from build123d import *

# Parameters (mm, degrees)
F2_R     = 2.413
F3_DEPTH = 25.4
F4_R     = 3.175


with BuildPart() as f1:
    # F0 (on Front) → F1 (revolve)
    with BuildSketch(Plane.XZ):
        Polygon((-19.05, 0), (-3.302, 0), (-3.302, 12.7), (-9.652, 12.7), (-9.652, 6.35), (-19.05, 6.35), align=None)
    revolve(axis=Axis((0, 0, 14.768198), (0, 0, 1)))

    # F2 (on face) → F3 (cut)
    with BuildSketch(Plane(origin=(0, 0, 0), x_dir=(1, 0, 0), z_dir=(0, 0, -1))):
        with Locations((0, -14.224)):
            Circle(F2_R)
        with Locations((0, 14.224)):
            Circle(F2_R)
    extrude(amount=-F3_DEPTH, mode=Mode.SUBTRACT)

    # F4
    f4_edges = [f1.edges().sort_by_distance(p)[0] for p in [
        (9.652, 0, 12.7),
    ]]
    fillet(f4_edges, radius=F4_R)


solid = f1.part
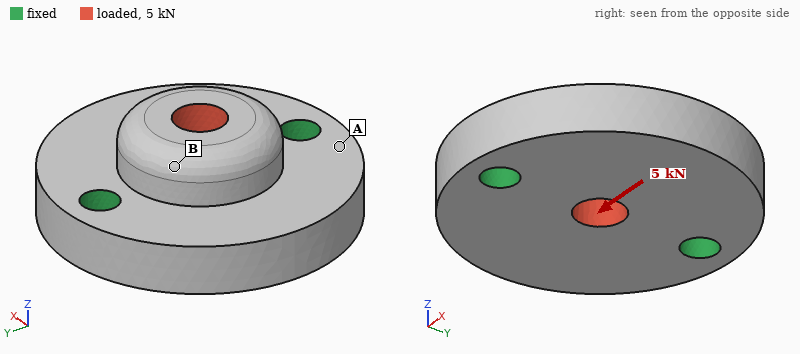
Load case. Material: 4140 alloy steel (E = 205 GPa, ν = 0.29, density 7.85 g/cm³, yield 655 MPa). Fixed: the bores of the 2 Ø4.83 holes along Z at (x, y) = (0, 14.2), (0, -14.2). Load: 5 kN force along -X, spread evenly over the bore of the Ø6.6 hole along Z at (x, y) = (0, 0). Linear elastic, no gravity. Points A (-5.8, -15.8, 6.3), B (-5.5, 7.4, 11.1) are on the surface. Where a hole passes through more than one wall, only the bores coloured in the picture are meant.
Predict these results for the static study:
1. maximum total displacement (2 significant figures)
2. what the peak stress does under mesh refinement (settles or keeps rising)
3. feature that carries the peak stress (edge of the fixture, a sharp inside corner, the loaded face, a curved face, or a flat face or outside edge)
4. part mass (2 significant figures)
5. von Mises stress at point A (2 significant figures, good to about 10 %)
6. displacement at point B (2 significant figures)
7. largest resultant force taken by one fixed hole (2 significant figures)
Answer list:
8.2 µm
keeps rising
edge of the fixture
65 g
35 MPa
5.9 µm
2.5 kN
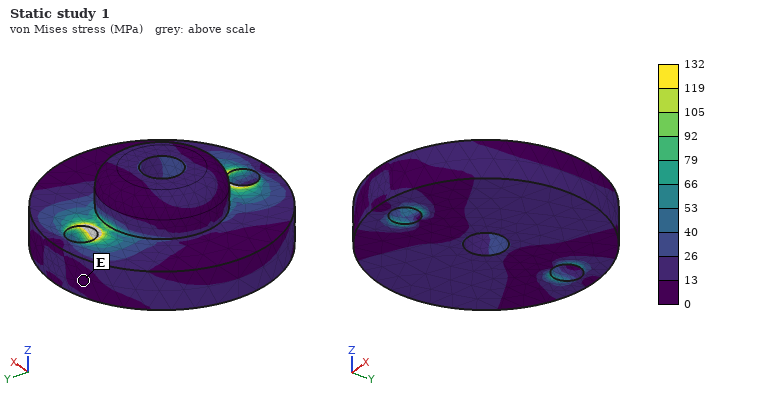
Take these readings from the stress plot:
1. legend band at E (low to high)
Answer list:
0 to 13 MPa
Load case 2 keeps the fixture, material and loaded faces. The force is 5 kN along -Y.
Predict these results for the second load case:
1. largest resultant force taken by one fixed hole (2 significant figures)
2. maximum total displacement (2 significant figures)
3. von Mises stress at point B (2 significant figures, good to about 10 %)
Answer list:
2.6 kN
2.8 µm
10.0 MPa
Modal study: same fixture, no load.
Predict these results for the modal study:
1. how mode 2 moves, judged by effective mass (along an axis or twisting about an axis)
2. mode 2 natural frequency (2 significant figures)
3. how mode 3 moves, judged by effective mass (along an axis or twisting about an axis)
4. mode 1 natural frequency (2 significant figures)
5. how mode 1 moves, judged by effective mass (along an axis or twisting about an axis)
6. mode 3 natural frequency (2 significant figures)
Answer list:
along Z
20 kHz
twisting about X
13 kHz
twisting about Y
36 kHz
